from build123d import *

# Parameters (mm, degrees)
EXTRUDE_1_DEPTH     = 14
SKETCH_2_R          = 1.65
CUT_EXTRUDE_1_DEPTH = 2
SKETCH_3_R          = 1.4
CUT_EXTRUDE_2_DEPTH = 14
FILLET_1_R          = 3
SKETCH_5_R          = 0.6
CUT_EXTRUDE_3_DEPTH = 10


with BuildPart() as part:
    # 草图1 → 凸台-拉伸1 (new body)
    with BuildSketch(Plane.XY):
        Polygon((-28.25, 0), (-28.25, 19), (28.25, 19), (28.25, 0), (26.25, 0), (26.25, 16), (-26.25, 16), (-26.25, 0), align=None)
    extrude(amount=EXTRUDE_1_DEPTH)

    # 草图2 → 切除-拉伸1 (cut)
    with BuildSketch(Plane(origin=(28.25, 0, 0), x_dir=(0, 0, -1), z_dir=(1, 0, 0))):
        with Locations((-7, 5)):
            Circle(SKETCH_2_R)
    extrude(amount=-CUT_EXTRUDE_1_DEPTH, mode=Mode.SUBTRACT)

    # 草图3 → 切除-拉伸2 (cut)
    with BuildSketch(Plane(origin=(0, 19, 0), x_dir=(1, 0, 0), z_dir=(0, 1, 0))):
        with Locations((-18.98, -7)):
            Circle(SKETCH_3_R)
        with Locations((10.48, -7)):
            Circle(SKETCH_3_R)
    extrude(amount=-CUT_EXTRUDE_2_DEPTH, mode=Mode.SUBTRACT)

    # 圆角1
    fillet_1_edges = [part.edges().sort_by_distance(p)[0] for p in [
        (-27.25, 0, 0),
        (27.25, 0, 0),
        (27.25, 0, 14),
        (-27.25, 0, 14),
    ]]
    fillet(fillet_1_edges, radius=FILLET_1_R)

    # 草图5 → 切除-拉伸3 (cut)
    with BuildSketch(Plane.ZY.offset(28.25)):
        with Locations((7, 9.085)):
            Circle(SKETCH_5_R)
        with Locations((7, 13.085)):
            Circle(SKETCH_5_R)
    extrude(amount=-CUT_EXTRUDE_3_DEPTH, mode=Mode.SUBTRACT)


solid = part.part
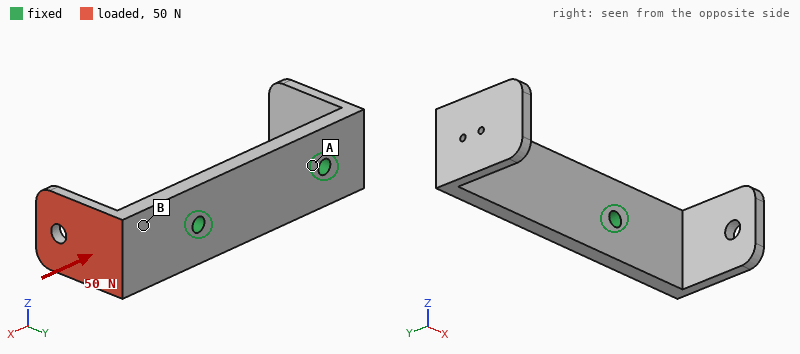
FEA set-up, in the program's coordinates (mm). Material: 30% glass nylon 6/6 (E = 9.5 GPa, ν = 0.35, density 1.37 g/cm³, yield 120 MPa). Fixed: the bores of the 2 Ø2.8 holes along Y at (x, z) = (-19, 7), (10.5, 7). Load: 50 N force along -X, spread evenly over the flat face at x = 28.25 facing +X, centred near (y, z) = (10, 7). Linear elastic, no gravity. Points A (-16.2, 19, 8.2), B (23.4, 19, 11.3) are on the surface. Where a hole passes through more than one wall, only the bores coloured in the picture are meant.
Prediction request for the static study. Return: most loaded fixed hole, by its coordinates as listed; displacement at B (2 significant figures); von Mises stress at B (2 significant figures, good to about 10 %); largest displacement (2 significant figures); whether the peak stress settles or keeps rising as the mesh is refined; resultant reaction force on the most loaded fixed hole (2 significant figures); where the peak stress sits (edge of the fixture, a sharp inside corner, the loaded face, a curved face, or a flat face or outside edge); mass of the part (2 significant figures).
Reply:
(10.5, 7)
0.11 mm
17 MPa
0.67 mm
keeps rising
45 N
edge of the fixture
4.4 g
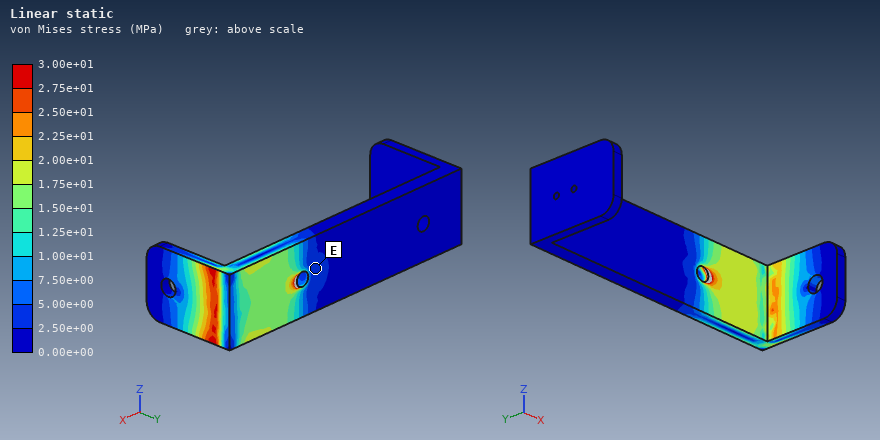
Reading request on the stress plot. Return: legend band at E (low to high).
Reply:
2.50e+00 to 5.00e+00 MPa
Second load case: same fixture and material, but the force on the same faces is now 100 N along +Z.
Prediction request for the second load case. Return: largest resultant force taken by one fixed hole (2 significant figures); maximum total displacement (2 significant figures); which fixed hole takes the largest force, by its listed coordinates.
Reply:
140 N
0.63 mm
(10.5, 7)
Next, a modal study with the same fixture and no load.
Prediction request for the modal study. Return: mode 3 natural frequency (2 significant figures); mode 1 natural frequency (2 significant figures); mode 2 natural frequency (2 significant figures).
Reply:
2700 Hz
1700 Hz
2400 Hz
